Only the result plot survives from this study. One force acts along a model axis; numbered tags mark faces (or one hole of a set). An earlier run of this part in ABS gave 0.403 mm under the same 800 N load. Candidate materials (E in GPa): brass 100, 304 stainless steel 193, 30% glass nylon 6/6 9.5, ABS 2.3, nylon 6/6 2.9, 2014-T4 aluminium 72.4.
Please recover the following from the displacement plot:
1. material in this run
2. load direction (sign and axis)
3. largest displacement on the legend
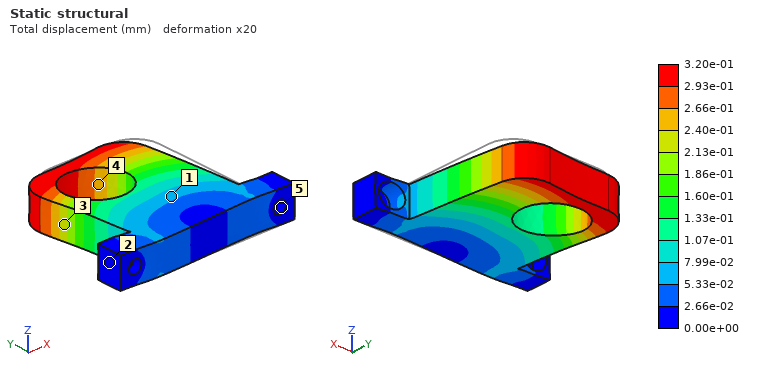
nylon 6/6
-X
3.20e-01 mm
